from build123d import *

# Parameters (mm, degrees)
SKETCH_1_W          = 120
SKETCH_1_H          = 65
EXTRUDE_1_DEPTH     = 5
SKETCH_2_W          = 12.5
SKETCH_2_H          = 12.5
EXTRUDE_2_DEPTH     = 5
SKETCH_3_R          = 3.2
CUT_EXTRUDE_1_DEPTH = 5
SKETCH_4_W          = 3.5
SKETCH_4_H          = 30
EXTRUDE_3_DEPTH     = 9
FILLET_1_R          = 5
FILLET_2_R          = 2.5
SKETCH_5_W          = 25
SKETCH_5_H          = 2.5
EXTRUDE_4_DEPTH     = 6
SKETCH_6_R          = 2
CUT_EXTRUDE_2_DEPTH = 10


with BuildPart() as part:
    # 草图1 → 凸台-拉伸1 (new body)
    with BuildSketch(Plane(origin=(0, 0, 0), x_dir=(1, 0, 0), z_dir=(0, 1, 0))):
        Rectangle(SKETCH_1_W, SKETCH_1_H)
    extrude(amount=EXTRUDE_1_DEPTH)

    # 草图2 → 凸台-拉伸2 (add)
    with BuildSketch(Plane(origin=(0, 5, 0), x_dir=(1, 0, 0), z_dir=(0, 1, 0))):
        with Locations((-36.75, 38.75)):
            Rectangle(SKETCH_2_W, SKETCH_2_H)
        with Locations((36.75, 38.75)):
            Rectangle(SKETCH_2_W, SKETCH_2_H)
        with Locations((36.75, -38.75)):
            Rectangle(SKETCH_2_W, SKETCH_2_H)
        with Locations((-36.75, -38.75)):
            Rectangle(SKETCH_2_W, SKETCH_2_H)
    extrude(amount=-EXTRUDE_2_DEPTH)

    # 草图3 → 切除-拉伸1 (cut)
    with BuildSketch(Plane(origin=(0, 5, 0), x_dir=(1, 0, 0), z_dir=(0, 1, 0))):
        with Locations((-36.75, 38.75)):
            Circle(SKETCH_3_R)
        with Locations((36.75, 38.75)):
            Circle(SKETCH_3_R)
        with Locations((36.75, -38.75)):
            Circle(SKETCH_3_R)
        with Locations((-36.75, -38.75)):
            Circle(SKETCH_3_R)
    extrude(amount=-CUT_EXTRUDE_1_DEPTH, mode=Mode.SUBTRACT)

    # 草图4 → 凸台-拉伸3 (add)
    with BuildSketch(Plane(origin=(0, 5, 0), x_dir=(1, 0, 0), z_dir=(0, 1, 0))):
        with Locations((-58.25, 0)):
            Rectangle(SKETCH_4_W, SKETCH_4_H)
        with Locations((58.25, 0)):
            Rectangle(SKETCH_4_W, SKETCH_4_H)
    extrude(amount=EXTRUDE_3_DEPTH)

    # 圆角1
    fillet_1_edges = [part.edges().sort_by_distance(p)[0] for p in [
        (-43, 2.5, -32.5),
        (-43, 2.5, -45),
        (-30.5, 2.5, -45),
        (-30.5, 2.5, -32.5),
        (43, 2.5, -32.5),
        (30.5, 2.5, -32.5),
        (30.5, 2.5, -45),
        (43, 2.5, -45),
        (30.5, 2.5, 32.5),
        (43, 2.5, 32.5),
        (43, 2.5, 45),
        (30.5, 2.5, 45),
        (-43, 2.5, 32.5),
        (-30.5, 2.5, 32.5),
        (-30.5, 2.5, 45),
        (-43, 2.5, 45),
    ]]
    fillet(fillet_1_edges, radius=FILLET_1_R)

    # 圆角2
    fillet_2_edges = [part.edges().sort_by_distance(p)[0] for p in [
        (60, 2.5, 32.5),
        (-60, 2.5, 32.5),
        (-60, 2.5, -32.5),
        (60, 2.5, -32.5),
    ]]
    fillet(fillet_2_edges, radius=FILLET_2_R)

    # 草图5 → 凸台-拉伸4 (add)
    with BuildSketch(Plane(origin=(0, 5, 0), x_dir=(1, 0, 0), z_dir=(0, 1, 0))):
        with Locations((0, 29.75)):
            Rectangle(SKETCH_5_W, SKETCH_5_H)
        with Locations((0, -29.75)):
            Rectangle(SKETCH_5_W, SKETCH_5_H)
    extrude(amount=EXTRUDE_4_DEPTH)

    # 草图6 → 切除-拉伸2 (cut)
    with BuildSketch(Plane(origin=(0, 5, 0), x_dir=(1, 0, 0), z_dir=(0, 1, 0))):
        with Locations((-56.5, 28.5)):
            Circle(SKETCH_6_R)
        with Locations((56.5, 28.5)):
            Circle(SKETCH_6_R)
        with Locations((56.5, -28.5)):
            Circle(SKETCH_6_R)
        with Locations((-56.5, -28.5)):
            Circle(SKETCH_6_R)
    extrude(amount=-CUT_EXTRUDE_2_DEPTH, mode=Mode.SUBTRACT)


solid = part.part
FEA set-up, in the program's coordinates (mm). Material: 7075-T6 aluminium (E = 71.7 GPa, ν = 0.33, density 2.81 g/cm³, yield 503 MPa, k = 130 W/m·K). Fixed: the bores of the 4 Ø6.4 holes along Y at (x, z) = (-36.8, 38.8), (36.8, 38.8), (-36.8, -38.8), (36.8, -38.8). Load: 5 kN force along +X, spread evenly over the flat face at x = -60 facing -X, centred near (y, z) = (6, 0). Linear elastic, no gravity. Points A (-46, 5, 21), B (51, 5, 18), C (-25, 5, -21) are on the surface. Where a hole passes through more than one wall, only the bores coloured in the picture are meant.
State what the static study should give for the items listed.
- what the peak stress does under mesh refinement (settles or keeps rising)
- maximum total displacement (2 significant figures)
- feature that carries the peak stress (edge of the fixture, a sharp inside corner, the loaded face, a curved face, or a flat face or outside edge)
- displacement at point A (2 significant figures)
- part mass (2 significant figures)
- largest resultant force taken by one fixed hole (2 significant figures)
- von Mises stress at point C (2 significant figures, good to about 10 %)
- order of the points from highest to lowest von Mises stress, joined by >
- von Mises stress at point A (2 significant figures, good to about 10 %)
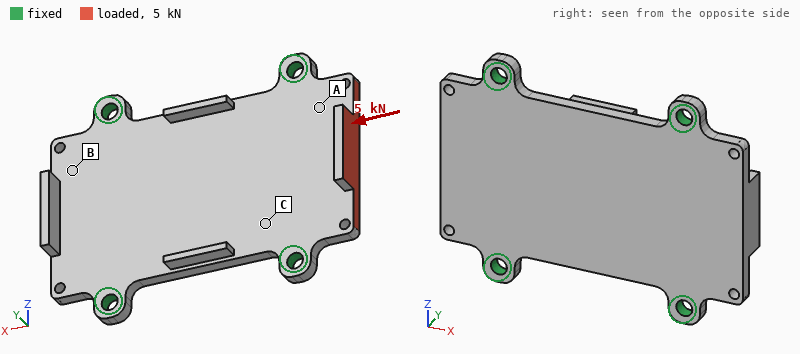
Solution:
keeps rising
0.27 mm
edge of the fixture
0.051 mm
120 g
1.6 kN
28 MPa
A > C > B
68 MPa
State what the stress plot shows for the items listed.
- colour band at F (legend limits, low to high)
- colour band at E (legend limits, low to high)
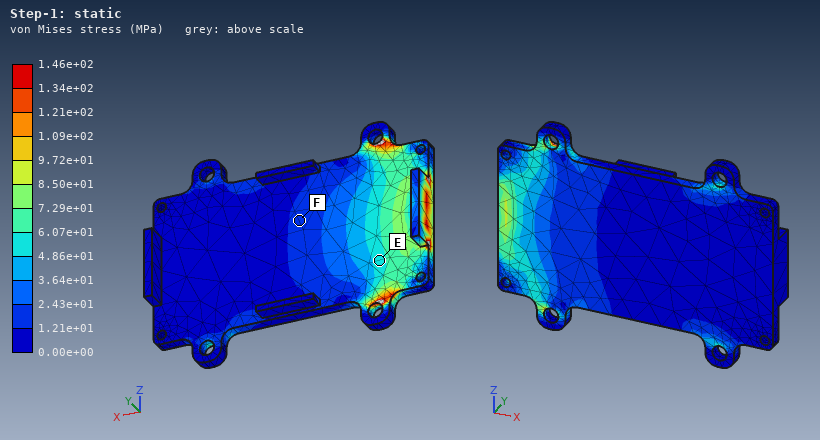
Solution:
1.21e+01 to 2.43e+01 MPa
4.86e+01 to 6.07e+01 MPa
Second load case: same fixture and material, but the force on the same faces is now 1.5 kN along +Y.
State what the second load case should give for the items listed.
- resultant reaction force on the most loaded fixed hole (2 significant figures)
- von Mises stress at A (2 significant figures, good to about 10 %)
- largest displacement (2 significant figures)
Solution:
870 N
89 MPa
0.41 mm
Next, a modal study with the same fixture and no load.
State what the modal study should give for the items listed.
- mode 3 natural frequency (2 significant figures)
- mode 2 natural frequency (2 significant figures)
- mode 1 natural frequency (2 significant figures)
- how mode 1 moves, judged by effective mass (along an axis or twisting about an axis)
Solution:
3200 Hz
3200 Hz
3000 Hz
along Y
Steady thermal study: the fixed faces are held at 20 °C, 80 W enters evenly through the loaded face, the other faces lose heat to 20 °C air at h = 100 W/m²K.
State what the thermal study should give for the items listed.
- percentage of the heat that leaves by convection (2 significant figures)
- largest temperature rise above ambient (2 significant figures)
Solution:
38 %
82 K
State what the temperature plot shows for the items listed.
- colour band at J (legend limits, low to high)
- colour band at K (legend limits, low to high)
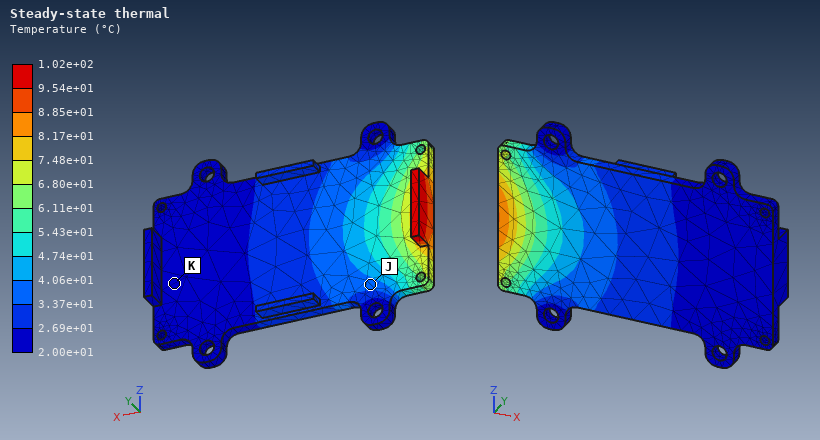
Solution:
3.37e+01 to 4.06e+01 °C
2.00e+01 to 2.69e+01 °C
